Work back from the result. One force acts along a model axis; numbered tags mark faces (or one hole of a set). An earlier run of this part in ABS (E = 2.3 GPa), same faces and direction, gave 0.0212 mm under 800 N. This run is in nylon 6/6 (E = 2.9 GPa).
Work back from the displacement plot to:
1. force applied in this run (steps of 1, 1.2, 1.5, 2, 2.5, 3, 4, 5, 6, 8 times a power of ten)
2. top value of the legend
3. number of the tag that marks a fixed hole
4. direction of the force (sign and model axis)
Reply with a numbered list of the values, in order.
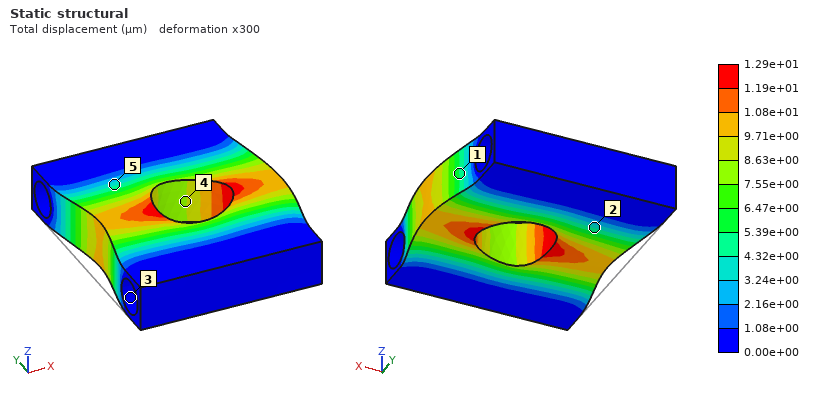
1. 600 N
2. 1.29e+01 µm
3. 3
4. +X
